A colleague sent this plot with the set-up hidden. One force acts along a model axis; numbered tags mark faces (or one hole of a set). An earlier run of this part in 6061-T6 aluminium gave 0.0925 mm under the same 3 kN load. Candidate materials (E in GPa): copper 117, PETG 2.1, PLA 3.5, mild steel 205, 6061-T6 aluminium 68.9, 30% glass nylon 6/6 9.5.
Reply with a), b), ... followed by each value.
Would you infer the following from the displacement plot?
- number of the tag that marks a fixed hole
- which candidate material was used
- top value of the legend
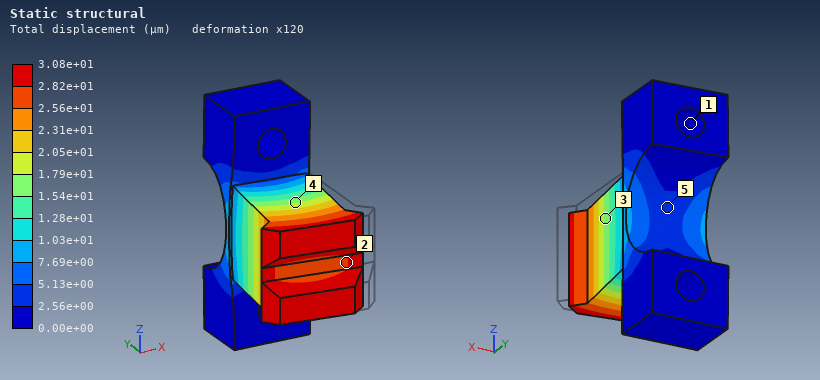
a) 1
b) mild steel
c) 3.08e+01 µm
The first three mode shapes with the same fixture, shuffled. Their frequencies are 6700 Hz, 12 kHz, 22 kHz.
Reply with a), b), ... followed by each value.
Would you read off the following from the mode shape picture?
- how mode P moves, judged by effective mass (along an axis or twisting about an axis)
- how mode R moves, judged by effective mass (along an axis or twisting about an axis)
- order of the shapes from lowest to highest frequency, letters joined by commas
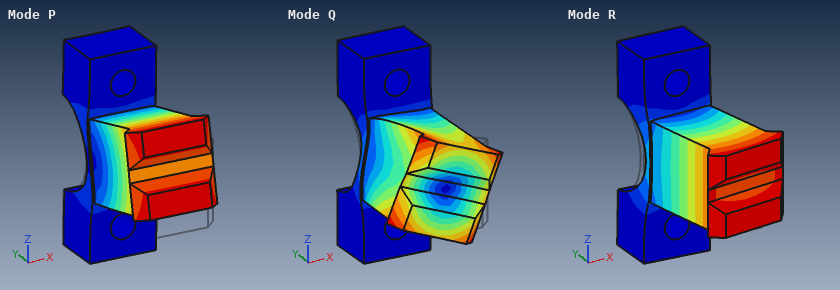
a) along Z
b) along X
c) R, P, Q
